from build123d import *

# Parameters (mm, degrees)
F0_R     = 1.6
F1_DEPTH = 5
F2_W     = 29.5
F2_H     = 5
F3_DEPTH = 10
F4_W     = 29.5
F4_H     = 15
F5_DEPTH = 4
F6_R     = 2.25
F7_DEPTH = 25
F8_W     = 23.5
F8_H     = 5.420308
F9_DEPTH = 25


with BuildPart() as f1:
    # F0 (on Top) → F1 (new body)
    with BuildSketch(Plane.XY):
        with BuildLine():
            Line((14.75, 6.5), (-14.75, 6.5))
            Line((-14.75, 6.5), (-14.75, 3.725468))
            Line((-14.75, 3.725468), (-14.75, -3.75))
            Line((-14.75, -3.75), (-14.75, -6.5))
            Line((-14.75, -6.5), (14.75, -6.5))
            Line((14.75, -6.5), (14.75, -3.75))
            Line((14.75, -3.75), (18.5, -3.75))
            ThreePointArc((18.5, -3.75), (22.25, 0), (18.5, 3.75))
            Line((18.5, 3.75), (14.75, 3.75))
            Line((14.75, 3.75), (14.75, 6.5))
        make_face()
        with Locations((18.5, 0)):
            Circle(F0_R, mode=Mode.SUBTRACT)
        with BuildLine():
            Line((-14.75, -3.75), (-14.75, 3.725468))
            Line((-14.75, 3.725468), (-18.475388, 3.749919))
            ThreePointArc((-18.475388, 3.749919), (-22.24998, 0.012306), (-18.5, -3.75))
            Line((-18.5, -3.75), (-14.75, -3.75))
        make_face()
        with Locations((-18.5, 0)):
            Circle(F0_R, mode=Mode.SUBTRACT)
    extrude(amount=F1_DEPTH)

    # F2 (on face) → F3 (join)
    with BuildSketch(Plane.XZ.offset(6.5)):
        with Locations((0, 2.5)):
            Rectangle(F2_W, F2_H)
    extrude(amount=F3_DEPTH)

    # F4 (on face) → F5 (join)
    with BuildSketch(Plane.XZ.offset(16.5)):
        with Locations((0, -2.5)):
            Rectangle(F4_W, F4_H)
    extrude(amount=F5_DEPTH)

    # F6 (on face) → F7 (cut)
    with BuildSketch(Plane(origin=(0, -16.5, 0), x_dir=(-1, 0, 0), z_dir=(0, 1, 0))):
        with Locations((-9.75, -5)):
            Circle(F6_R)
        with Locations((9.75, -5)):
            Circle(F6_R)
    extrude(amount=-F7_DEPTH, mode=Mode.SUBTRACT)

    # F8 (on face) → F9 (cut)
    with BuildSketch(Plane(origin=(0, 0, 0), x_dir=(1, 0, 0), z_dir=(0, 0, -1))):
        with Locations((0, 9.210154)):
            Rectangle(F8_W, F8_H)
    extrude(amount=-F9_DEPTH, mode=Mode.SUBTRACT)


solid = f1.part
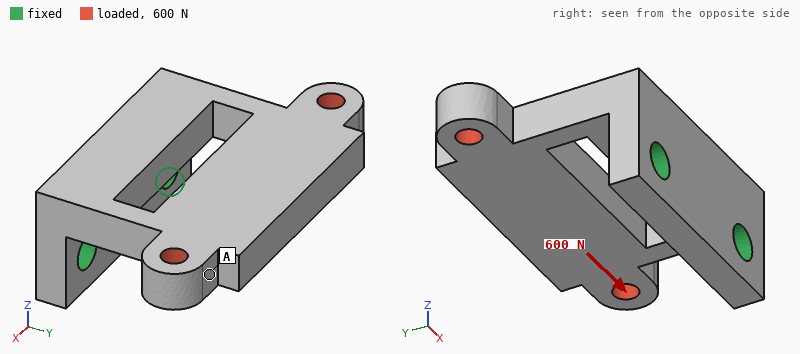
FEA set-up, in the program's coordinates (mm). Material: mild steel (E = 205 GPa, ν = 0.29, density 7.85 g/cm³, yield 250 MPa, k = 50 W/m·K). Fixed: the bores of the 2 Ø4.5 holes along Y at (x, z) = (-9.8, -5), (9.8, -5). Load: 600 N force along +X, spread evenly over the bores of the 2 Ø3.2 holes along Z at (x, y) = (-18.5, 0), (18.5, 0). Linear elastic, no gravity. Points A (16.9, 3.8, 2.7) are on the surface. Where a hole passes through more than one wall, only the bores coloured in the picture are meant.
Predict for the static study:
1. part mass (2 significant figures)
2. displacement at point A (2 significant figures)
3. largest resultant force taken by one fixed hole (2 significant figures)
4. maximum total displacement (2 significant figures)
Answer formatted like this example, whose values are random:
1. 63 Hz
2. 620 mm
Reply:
1. 38 g
2. 20 µm
3. 600 N
4. 21 µm
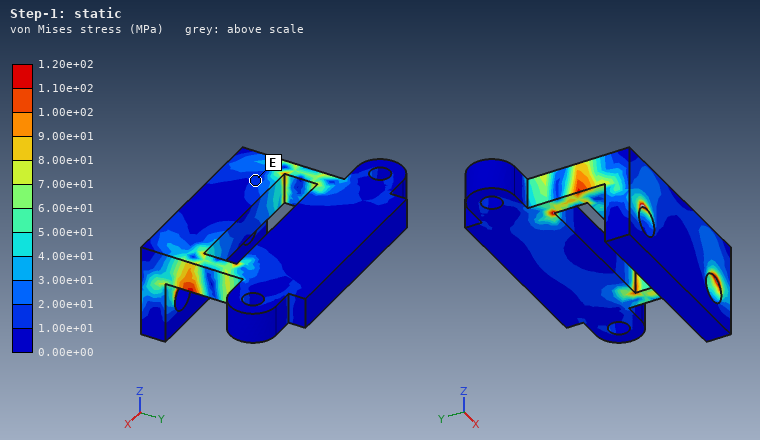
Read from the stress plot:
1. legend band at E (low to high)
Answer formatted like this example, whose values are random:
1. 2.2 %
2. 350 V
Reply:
1. 1.00e+01 to 2.00e+01 MPa
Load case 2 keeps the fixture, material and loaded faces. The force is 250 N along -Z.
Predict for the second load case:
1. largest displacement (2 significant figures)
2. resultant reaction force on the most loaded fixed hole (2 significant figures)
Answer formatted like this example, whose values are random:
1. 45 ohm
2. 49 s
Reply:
1. 64 µm
2. 130 N
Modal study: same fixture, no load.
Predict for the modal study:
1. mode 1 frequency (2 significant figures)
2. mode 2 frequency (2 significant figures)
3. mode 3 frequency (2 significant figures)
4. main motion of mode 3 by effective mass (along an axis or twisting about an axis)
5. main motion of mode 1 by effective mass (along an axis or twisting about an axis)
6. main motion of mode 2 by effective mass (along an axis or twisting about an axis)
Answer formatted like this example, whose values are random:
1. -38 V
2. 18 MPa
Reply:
1. 2700 Hz
2. 6100 Hz
3. 7500 Hz
4. along X
5. along Z
6. along X
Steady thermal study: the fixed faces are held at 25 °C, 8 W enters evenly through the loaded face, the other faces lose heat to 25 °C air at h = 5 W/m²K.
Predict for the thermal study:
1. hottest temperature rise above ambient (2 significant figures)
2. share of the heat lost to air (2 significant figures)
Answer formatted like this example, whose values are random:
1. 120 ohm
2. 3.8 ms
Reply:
1. 81 K
2. 7.0 %
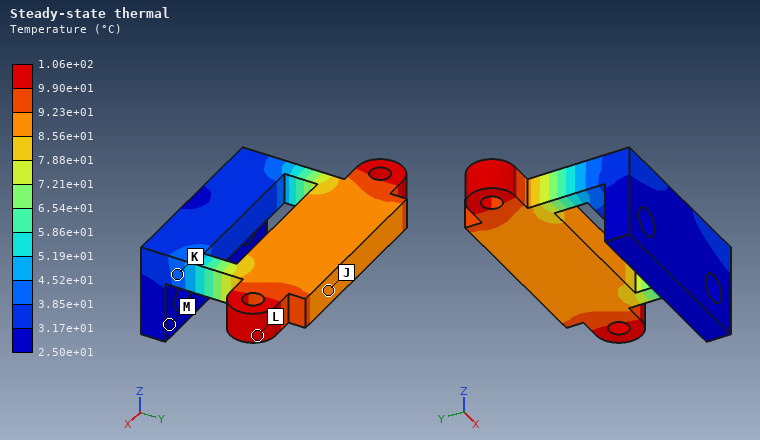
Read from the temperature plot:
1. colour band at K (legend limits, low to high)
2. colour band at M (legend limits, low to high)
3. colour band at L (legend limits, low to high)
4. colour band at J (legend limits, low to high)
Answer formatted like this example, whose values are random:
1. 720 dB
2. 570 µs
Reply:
1. 3.85e+01 to 4.52e+01 °C
2. 2.50e+01 to 3.17e+01 °C
3. 9.90e+01 to 1.06e+02 °C
4. 8.56e+01 to 9.23e+01 °C
